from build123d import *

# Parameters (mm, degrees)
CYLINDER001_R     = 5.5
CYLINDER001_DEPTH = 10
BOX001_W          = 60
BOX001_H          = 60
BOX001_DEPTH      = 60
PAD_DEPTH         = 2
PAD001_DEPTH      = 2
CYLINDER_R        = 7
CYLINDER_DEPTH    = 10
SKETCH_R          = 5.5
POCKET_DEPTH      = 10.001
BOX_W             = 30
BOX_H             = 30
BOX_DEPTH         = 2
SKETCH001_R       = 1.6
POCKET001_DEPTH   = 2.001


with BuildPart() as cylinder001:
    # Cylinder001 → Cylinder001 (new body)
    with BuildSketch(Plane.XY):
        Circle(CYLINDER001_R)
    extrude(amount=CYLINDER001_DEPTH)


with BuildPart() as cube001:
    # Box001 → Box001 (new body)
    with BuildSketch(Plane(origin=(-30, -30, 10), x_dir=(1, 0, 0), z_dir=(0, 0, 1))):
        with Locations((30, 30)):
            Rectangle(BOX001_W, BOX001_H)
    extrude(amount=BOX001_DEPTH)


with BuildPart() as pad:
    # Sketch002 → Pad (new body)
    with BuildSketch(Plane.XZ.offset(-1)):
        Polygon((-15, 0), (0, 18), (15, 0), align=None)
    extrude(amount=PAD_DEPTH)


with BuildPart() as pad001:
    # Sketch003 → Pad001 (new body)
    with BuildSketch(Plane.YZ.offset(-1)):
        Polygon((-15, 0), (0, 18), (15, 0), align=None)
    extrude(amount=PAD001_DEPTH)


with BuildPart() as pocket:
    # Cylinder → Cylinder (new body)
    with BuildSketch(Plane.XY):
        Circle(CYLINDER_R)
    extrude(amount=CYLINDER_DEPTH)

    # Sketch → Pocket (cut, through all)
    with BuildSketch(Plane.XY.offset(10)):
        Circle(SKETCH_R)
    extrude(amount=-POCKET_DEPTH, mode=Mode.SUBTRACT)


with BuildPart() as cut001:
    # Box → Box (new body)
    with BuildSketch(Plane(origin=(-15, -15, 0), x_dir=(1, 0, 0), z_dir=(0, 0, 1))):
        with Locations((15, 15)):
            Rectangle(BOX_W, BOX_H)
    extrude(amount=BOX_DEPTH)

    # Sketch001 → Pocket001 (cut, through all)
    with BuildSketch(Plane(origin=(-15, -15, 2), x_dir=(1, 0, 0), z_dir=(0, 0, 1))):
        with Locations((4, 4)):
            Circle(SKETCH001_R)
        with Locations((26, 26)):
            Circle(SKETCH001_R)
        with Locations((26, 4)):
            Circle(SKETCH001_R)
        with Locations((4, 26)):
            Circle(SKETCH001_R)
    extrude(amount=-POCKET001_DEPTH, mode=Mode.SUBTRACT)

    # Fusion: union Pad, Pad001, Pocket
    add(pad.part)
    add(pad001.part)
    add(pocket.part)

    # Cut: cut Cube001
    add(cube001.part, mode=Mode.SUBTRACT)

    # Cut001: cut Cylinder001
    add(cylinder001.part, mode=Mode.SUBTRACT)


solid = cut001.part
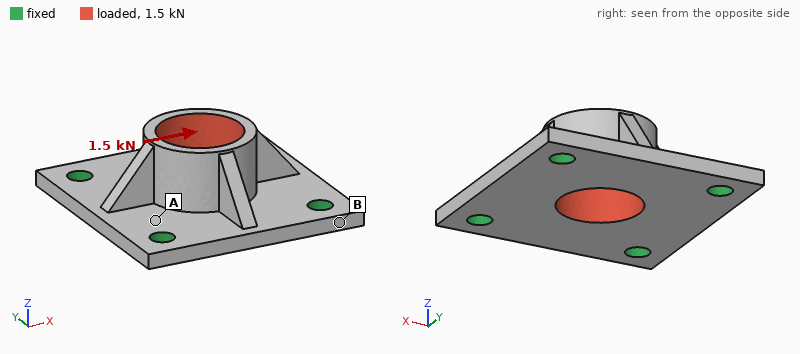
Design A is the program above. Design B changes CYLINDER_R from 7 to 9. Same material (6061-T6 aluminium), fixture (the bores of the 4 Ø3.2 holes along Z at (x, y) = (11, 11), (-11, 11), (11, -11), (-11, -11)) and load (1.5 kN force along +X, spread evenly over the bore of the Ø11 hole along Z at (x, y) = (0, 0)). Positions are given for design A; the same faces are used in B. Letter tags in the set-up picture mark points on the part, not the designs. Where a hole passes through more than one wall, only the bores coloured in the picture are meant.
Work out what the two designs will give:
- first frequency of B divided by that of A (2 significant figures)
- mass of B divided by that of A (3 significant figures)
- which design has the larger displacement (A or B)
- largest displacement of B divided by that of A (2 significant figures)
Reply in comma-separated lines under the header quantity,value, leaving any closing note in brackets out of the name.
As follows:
quantity,value
first frequency of B divided by that of A,0.97
mass of B divided by that of A,1.32
which design has the larger displacement,A
largest displacement of B divided by that of A,0.66
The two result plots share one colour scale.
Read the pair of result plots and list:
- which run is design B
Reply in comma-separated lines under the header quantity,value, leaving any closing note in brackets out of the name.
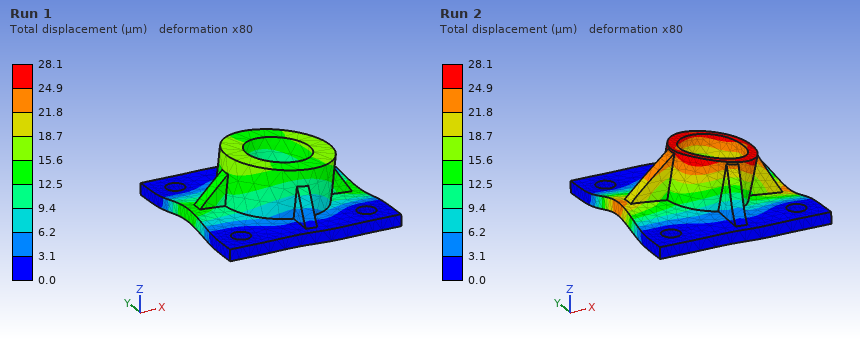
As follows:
quantity,value
which run is design B,Run 1
